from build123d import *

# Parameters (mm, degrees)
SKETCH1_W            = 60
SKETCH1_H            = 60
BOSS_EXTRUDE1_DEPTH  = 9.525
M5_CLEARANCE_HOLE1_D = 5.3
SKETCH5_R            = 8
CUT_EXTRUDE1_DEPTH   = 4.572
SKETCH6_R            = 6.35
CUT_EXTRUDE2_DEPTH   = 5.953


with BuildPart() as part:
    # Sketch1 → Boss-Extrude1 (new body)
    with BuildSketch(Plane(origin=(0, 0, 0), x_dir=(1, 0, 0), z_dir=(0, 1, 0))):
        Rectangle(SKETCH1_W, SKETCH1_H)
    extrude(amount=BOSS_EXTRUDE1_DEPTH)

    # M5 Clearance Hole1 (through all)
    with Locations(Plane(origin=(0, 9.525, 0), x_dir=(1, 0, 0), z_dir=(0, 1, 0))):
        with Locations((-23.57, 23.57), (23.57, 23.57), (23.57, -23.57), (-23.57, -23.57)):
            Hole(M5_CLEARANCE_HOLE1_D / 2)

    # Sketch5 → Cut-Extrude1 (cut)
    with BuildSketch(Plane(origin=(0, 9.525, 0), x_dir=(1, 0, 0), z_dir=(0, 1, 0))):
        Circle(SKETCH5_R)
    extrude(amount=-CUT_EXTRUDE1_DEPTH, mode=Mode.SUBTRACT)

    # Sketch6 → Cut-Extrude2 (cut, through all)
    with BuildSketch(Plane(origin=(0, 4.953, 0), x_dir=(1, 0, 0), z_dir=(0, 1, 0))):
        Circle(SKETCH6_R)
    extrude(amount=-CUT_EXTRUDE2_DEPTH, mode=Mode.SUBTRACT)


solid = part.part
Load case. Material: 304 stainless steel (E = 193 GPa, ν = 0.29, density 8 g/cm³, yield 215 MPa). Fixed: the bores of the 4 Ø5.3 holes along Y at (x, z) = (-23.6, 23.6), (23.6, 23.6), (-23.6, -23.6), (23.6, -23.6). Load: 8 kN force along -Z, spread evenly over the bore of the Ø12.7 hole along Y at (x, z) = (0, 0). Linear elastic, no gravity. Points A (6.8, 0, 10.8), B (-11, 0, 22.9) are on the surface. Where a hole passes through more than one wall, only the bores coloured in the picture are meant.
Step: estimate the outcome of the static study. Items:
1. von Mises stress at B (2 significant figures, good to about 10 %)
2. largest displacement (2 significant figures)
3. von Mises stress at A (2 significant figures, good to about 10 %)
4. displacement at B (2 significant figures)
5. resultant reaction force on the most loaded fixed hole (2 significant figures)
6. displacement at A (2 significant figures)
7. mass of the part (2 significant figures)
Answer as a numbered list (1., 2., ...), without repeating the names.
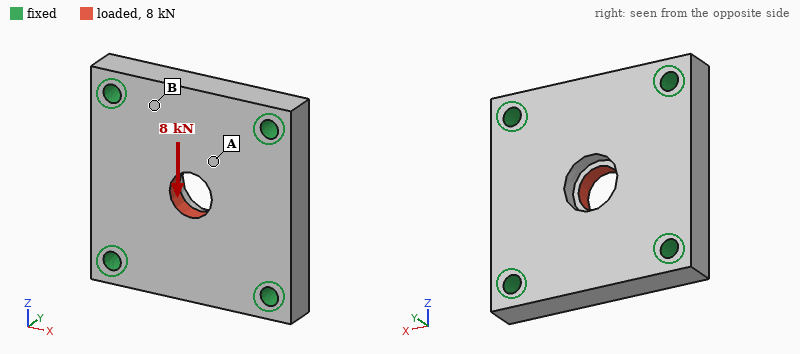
1. 11 MPa
2. 4.2 µm
3. 28 MPa
4. 1.6 µm
5. 2.2 kN
6. 2.5 µm
7. 260 g
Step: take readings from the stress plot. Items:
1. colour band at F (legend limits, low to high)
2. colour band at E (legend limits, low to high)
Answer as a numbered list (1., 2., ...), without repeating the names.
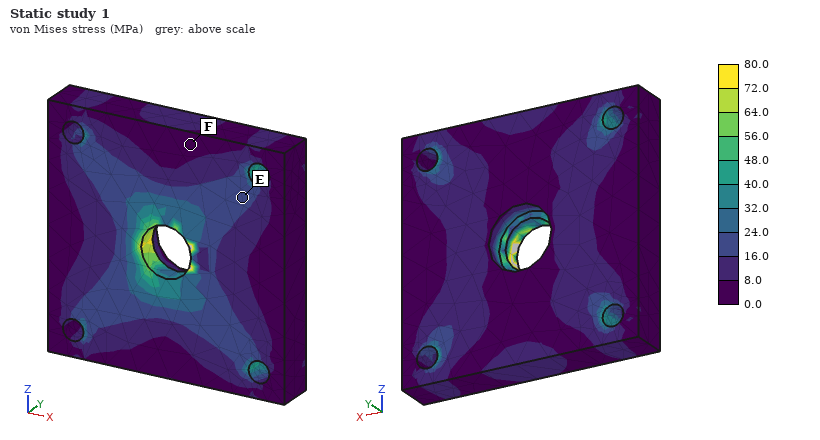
1. 0.0 to 8.0 MPa
2. 16.0 to 24.0 MPa
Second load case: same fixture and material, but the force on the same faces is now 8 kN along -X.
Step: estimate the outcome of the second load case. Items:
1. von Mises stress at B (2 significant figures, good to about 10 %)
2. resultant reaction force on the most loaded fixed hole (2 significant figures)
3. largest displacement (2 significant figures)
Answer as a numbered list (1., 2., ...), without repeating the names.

1. 10 MPa
2. 2.2 kN
3. 4.2 µm
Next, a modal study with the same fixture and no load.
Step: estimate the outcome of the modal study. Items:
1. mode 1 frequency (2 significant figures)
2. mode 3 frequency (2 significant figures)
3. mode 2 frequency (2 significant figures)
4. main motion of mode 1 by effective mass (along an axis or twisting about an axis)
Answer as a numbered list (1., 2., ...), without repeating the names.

1. 13 kHz
2. 19 kHz
3. 19 kHz
4. along Y
